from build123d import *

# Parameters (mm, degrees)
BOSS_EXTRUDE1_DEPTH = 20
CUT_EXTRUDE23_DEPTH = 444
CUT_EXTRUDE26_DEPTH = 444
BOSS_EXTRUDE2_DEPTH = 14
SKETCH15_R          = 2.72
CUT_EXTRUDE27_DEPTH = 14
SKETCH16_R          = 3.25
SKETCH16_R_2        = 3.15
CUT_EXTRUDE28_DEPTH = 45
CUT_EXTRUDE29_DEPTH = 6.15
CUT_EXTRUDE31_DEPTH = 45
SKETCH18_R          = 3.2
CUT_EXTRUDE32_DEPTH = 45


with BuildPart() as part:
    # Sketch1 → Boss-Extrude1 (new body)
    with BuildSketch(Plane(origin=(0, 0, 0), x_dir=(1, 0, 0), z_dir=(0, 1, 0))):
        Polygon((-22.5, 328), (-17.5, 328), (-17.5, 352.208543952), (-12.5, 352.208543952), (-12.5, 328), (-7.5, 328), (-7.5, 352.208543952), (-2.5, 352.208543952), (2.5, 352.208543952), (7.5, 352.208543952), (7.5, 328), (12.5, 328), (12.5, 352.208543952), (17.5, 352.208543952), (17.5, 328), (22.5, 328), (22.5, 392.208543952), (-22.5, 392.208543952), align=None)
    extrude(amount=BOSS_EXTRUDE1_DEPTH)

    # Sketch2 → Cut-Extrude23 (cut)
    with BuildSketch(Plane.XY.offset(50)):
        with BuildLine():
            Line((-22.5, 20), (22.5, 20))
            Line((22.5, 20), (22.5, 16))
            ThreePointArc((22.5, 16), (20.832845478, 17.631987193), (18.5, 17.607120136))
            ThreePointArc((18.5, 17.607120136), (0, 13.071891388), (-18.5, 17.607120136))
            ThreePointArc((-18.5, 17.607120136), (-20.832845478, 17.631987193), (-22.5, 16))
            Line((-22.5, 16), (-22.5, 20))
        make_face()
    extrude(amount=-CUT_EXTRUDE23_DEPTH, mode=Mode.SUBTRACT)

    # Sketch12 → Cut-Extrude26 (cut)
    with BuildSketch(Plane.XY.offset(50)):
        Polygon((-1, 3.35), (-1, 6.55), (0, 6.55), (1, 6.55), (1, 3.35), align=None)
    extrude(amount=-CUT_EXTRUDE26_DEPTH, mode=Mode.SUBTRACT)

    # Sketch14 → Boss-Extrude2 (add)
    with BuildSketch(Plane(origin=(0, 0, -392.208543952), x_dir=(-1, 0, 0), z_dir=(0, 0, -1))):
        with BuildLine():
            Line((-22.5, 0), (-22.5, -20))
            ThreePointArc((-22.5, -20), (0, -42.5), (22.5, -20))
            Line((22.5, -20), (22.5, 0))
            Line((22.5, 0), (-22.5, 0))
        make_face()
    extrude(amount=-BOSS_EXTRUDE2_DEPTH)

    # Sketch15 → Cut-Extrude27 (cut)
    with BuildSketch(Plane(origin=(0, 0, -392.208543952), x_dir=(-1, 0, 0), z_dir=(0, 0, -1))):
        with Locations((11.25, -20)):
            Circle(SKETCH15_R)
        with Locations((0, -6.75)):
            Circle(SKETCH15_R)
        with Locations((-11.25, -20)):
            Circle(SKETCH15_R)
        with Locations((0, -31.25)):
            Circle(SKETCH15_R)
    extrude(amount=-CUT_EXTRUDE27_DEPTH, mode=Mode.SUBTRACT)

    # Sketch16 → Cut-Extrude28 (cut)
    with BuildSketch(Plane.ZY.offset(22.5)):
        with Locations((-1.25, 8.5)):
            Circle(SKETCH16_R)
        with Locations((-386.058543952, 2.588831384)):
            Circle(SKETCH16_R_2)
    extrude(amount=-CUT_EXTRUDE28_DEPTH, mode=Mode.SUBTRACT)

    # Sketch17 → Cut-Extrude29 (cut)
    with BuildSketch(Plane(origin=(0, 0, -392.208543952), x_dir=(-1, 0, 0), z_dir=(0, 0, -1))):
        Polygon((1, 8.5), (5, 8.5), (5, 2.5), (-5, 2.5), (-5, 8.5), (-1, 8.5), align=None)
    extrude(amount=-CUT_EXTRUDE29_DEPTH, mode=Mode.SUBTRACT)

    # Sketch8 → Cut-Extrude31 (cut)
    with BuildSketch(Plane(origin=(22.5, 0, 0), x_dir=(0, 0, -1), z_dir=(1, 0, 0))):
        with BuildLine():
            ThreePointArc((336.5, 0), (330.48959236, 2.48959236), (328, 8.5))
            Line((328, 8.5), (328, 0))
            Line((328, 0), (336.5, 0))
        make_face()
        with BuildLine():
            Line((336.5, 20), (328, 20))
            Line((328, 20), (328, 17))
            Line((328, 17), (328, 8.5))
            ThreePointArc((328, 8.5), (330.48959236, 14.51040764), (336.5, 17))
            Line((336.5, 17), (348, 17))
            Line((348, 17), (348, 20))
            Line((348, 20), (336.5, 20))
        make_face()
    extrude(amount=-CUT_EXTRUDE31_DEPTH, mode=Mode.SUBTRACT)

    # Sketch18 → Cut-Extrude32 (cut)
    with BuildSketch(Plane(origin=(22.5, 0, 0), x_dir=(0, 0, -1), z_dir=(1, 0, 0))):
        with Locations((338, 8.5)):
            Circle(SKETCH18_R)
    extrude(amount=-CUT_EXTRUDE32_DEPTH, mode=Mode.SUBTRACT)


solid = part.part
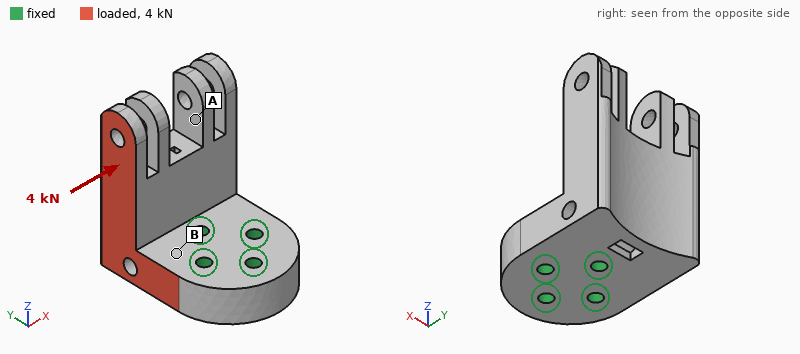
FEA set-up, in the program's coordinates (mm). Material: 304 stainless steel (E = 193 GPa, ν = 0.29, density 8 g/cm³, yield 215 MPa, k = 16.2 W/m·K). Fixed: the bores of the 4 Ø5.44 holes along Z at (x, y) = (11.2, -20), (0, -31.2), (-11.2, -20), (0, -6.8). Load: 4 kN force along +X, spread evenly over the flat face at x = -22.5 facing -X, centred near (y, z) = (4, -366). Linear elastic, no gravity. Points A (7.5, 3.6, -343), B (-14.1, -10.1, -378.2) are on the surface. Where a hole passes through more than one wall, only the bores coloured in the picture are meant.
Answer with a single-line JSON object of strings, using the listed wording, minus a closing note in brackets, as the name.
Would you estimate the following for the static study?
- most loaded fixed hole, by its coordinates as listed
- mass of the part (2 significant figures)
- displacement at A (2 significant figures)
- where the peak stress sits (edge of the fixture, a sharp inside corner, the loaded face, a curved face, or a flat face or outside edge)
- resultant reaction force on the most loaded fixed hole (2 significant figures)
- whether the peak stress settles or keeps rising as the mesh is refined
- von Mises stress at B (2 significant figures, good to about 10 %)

{"most loaded fixed hole, by its coordinates as listed": "(0, -6.8)", "mass of the part": "430 g", "displacement at A": "0.019 mm", "where the peak stress sits": "edge of the fixture", "resultant reaction force on the most loaded fixed hole": "3.8 kN", "whether the peak stress settles or keeps rising as the mesh is refined": "keeps rising", "von Mises stress at B": "23 MPa"}
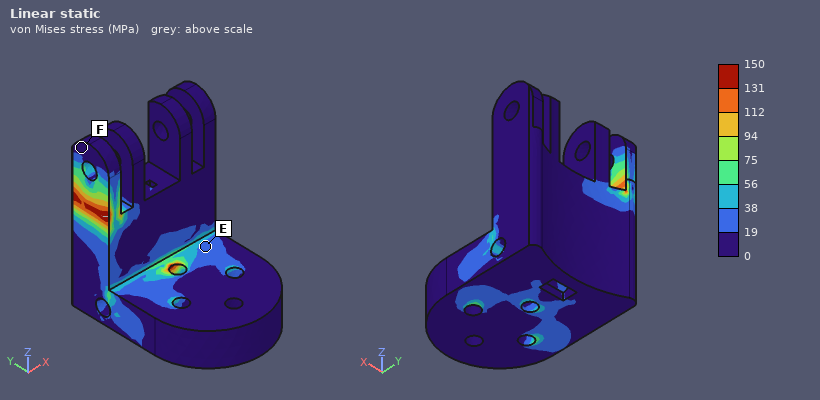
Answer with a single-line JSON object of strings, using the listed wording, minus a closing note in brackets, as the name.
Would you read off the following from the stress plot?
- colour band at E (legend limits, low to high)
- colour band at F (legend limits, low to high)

{"colour band at E": "19 to 38 MPa", "colour band at F": "0 to 19 MPa"}
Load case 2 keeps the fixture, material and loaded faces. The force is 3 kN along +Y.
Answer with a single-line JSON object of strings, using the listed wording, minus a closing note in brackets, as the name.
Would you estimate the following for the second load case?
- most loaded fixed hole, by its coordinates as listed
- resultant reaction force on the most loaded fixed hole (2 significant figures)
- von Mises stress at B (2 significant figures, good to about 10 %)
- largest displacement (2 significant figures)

{"most loaded fixed hole, by its coordinates as listed": "(-11.2, -20)", "resultant reaction force on the most loaded fixed hole": "2.7 kN", "von Mises stress at B": "43 MPa", "largest displacement": "77 µm"}
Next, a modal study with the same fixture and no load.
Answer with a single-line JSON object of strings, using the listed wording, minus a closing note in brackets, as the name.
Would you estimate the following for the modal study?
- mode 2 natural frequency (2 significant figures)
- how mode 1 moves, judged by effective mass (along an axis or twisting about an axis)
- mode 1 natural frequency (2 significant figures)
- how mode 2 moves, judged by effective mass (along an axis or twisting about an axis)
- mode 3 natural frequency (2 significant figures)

{"mode 2 natural frequency": "4000 Hz", "how mode 1 moves, judged by effective mass": "along Y", "mode 1 natural frequency": "3000 Hz", "how mode 2 moves, judged by effective mass": "along X", "mode 3 natural frequency": "6100 Hz"}
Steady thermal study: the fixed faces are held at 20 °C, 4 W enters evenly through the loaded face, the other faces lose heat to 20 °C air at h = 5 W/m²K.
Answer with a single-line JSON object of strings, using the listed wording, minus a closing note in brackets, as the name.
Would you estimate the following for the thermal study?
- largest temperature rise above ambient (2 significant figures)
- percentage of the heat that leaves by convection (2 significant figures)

{"largest temperature rise above ambient": "26 K", "percentage of the heat that leaves by convection": "11 %"}
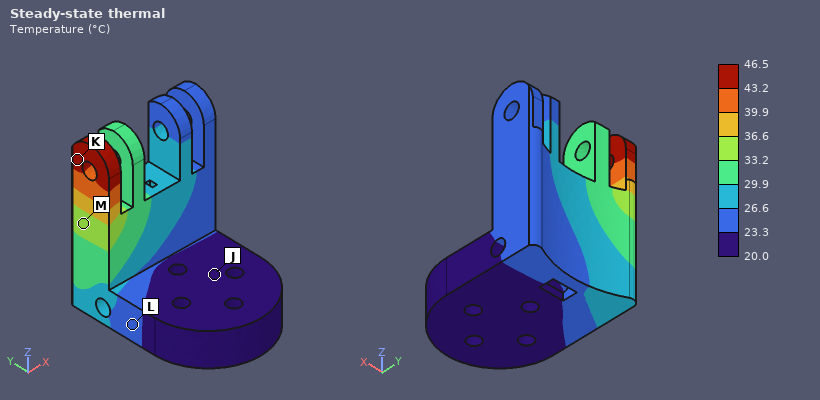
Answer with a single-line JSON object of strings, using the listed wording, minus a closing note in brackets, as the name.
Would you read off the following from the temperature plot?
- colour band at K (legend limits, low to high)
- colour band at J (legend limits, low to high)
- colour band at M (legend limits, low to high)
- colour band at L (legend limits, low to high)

{"colour band at K": "43.2 to 46.5 °C", "colour band at J": "20.0 to 23.3 °C", "colour band at M": "33.2 to 36.6 °C", "colour band at L": "23.3 to 26.6 °C"}
